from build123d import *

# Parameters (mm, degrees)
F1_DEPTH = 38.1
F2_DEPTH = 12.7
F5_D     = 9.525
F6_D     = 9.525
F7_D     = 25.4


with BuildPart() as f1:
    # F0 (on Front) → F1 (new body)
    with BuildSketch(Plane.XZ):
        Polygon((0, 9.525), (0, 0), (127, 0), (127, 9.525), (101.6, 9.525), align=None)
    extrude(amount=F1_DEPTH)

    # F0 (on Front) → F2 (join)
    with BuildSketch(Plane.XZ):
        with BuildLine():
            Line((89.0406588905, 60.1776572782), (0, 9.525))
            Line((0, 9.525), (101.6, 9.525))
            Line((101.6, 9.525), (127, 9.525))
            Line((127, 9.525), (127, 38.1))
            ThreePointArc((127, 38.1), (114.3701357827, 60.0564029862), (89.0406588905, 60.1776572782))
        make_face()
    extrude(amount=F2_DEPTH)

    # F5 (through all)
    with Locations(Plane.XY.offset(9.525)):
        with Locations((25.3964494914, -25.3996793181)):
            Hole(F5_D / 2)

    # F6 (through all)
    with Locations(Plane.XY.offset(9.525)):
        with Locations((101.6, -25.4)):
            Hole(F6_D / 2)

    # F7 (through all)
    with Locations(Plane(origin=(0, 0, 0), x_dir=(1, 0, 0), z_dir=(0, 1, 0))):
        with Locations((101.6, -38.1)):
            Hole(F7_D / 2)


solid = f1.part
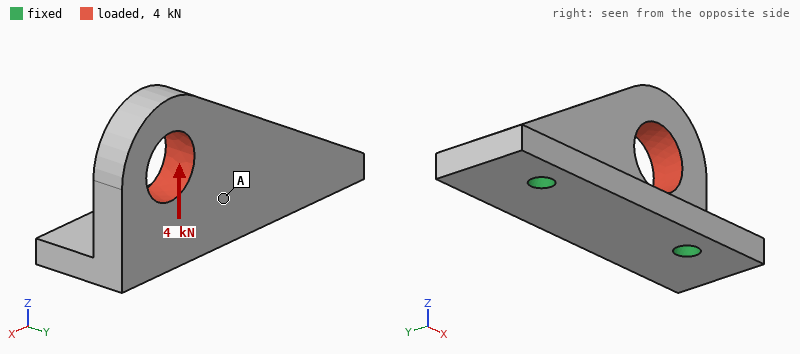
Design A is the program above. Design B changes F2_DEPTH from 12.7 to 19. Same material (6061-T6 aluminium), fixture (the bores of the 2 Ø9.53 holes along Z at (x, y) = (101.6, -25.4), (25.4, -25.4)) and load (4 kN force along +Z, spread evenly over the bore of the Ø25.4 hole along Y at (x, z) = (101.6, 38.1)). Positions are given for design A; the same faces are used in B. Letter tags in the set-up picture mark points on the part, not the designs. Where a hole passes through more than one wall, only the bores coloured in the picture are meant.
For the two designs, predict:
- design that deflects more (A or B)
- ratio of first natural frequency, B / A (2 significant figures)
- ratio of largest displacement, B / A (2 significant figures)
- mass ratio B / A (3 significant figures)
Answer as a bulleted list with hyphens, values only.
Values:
- A
- 1.0
- 0.63
- 1.25
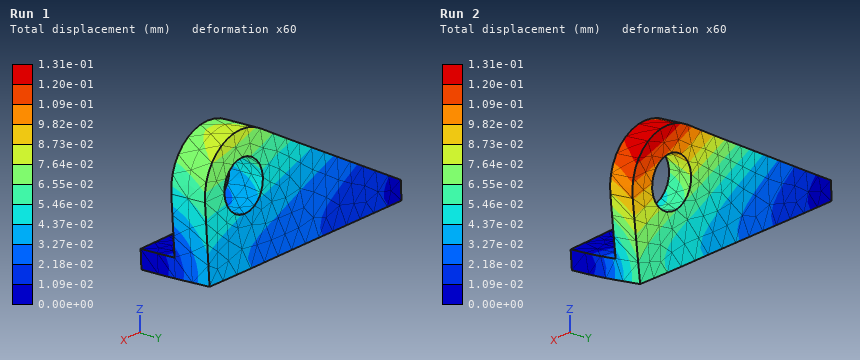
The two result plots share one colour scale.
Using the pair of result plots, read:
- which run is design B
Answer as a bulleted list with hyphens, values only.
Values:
- Run 1
